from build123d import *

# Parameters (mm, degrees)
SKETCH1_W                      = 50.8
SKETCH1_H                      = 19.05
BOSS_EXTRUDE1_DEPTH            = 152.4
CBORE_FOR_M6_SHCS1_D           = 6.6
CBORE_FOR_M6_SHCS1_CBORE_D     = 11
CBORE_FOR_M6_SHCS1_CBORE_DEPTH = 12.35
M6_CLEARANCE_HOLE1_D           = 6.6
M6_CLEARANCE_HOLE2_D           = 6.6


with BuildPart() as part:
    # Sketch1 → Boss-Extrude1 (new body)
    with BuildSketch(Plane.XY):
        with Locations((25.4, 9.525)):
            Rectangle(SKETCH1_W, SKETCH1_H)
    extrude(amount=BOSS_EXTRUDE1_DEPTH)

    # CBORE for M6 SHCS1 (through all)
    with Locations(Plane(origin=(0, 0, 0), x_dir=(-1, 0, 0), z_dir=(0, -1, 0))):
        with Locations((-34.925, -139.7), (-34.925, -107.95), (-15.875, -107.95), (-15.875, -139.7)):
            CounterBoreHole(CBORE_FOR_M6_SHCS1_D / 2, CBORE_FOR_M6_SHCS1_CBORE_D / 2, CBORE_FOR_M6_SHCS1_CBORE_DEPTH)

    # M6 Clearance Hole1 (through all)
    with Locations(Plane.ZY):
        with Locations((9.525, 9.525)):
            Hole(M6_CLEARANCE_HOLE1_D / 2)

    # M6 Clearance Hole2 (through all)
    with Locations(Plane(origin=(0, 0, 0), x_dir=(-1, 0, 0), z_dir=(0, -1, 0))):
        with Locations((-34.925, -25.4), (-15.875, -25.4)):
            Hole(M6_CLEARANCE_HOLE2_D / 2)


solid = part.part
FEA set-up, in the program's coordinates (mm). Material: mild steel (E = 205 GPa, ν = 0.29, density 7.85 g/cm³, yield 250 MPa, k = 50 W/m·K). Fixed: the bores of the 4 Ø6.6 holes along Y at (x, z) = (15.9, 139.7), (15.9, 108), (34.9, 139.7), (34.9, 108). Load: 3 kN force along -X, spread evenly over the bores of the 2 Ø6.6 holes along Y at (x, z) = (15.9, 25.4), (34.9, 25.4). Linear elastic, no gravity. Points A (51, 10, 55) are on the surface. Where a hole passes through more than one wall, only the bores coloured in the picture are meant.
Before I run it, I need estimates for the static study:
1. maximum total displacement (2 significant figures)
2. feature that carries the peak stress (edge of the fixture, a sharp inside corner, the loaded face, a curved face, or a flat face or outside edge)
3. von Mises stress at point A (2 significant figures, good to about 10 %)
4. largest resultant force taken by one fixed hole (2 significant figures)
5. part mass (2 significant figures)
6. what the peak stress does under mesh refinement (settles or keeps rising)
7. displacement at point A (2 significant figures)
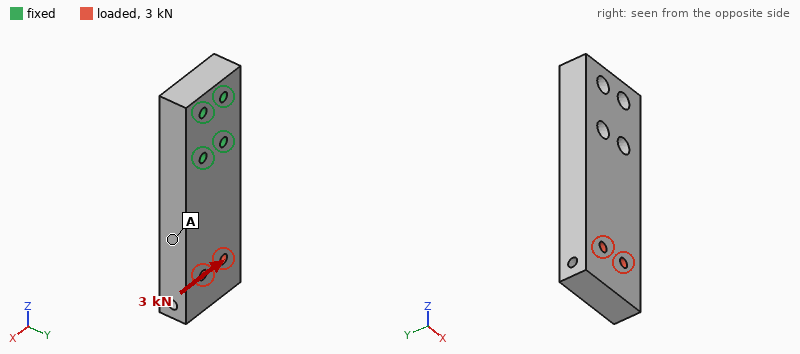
38 µm
edge of the fixture
11 MPa
5.7 kN
1.1 kg
keeps rising
18 µm
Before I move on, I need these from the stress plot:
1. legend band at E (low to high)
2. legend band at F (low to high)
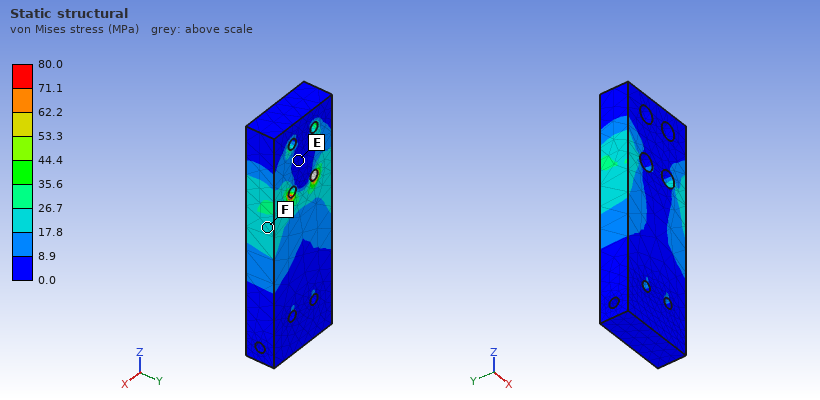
0.0 to 8.9 MPa
17.8 to 26.7 MPa
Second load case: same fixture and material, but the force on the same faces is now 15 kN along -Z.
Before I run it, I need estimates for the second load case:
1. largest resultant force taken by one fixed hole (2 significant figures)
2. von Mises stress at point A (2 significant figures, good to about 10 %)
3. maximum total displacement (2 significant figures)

5.4 kN
15 MPa
24 µm
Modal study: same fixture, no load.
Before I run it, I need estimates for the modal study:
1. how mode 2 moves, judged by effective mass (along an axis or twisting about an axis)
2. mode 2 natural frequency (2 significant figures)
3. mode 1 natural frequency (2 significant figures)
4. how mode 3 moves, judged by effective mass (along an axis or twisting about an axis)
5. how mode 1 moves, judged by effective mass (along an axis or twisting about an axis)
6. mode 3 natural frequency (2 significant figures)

along X
2500 Hz
1100 Hz
twisting about Z
along Y
4300 Hz
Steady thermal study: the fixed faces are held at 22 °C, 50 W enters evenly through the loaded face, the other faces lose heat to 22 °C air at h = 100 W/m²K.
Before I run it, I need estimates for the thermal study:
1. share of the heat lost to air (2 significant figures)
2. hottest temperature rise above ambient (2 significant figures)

75 %
40 K
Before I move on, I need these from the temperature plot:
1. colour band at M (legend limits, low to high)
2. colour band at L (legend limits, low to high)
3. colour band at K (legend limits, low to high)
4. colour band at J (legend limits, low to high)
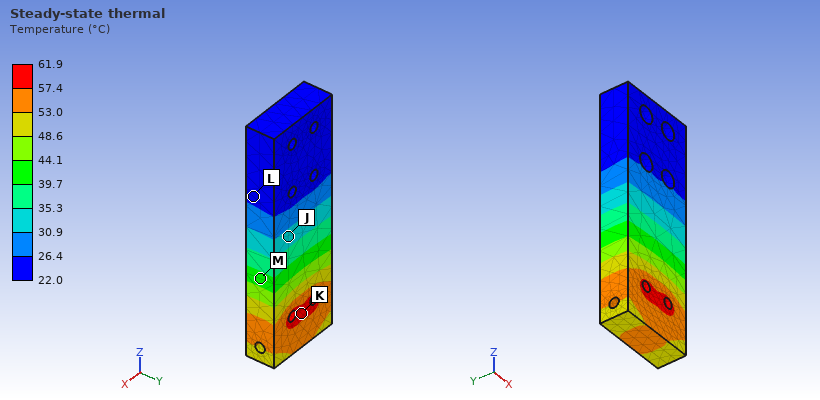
39.7 to 44.1 °C
22.0 to 26.4 °C
57.4 to 61.9 °C
30.9 to 35.3 °C
